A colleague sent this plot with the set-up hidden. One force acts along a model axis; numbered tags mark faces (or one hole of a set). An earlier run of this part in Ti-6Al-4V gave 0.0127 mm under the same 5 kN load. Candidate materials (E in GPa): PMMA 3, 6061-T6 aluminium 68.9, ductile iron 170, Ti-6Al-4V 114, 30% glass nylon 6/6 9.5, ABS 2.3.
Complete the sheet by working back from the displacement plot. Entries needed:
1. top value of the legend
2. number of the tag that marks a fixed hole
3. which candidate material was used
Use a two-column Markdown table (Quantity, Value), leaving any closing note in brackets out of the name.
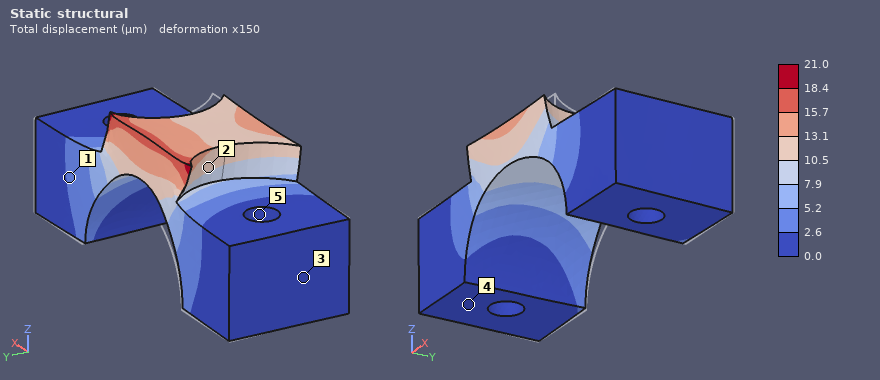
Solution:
| Quantity | Value |
|---|---|
| top value of the legend | 21.0 µm |
| number of the tag that marks a fixed hole | 5 |
| which candidate material was used | 6061-T6 aluminium |
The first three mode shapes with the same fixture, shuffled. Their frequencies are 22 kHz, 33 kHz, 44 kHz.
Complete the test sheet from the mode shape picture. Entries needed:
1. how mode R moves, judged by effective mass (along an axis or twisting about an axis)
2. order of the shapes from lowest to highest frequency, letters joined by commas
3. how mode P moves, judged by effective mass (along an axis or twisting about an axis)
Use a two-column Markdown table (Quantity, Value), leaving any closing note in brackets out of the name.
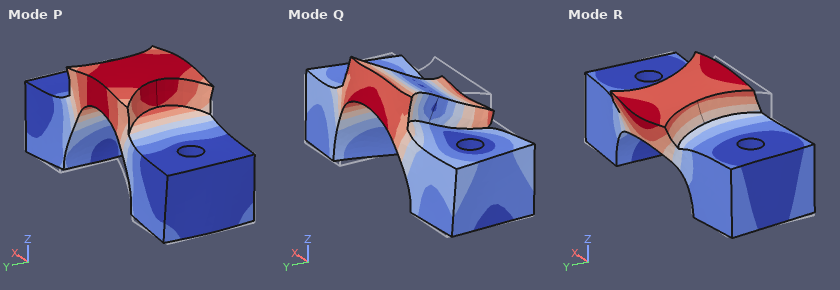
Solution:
| Quantity | Value |
|---|---|
| how mode R moves, judged by effective mass | along Y |
| order of the shapes from lowest to highest frequency, letters joined by commas | R, P, Q |
| how mode P moves, judged by effective mass | along Z |
